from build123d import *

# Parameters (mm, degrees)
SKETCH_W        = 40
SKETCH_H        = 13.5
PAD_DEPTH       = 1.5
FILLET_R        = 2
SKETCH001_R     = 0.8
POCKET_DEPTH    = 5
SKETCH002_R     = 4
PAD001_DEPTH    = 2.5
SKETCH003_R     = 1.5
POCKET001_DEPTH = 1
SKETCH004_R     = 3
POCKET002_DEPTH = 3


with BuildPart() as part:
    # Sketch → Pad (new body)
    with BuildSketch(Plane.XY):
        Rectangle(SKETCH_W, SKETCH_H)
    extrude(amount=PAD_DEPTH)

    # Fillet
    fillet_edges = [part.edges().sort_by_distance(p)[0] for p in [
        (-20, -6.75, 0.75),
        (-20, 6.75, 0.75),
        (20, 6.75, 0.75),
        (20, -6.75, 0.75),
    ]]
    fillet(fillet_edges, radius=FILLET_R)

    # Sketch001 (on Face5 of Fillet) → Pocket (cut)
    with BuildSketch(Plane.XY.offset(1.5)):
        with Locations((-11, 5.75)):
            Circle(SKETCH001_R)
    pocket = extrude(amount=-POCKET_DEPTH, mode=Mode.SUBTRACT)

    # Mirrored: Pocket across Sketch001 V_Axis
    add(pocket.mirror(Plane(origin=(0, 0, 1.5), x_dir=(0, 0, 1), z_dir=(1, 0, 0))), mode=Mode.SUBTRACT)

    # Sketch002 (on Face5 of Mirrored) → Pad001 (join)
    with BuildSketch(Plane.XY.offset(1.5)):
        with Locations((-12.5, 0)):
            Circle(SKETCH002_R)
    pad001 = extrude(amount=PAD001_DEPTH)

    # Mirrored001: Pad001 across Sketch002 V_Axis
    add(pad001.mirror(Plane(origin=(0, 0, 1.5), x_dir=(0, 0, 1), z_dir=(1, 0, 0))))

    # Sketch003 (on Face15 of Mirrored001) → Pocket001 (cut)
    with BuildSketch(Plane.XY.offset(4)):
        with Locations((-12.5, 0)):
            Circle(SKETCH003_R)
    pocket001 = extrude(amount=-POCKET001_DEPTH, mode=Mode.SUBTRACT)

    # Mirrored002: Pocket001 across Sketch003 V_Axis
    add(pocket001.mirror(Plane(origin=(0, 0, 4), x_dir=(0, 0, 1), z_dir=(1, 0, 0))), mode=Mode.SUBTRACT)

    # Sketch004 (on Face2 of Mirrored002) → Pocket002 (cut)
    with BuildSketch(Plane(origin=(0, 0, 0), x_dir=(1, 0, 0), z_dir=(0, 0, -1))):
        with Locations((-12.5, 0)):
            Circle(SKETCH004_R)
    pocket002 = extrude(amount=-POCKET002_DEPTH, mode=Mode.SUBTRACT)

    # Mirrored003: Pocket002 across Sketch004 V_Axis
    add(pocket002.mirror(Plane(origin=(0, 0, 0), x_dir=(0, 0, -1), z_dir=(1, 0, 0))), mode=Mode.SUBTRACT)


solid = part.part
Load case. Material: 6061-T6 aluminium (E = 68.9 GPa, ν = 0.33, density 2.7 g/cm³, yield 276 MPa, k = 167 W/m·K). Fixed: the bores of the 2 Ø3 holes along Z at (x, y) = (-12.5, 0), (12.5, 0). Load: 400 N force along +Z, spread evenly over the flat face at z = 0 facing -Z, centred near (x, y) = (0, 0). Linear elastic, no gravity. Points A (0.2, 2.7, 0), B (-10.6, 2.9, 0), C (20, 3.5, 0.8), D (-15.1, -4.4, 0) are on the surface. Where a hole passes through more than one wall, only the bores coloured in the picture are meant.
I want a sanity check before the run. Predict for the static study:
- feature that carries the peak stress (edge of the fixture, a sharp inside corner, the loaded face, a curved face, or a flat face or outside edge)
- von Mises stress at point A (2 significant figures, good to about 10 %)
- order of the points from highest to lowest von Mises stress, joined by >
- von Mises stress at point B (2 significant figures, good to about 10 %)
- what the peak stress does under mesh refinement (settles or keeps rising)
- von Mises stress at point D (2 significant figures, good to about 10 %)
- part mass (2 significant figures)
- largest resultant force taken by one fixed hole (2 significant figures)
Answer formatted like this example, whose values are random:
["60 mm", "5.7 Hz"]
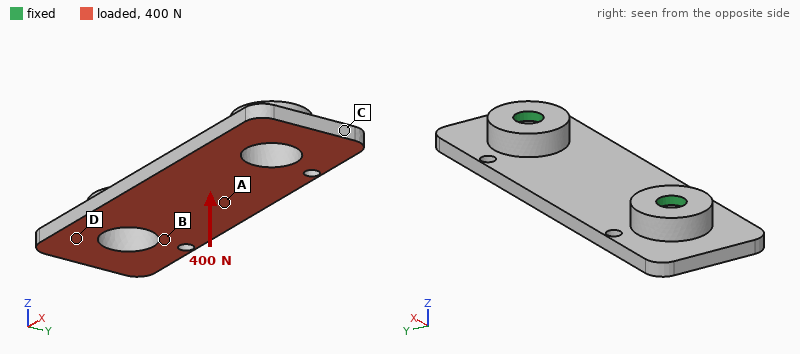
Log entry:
["edge of the fixture", "46 MPa", "A > B > D > C", "36 MPa", "keeps rising", "16 MPa", "2.3 g", "220 N"]
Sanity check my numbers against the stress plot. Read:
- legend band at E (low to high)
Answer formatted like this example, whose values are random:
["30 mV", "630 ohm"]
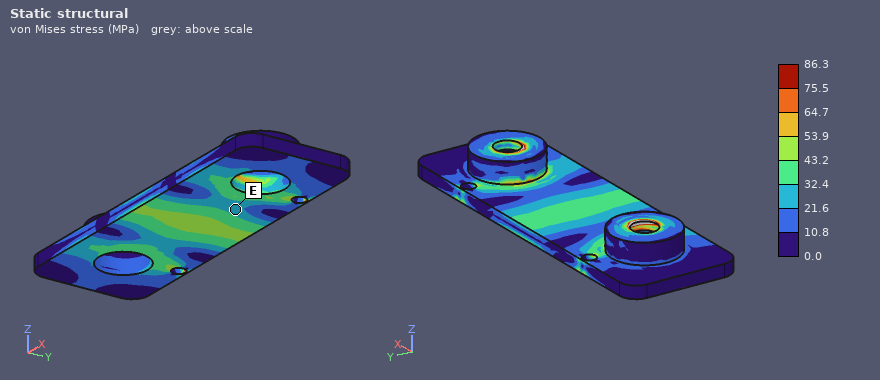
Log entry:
["21.6 to 32.4 MPa"]
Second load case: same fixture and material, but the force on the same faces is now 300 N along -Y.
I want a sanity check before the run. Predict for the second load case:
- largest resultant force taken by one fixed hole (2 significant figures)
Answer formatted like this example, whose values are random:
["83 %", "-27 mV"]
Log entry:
["150 N"]
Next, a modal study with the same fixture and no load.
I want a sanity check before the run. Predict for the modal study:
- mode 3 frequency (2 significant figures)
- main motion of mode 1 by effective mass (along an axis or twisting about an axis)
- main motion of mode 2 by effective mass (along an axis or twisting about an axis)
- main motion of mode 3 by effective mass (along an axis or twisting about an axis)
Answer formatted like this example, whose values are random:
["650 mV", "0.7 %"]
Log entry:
["18 kHz", "along Y", "along Z", "along X"]
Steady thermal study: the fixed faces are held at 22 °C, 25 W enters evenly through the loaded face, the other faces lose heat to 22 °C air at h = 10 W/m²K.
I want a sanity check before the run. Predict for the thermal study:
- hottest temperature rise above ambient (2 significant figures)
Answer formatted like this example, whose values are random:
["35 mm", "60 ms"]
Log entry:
["29 K"]
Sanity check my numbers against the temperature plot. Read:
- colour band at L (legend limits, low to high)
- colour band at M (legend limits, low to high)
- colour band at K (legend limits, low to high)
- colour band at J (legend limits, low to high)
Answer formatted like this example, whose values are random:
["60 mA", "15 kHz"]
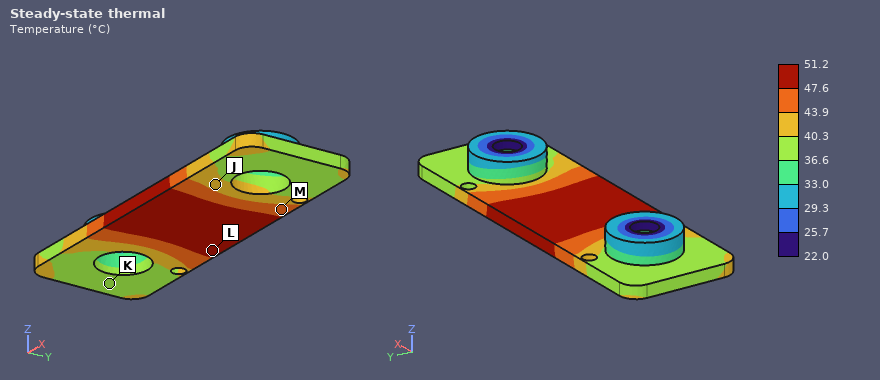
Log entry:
["47.6 to 51.2 °C", "43.9 to 47.6 °C", "36.6 to 40.3 °C", "40.3 to 43.9 °C"]
